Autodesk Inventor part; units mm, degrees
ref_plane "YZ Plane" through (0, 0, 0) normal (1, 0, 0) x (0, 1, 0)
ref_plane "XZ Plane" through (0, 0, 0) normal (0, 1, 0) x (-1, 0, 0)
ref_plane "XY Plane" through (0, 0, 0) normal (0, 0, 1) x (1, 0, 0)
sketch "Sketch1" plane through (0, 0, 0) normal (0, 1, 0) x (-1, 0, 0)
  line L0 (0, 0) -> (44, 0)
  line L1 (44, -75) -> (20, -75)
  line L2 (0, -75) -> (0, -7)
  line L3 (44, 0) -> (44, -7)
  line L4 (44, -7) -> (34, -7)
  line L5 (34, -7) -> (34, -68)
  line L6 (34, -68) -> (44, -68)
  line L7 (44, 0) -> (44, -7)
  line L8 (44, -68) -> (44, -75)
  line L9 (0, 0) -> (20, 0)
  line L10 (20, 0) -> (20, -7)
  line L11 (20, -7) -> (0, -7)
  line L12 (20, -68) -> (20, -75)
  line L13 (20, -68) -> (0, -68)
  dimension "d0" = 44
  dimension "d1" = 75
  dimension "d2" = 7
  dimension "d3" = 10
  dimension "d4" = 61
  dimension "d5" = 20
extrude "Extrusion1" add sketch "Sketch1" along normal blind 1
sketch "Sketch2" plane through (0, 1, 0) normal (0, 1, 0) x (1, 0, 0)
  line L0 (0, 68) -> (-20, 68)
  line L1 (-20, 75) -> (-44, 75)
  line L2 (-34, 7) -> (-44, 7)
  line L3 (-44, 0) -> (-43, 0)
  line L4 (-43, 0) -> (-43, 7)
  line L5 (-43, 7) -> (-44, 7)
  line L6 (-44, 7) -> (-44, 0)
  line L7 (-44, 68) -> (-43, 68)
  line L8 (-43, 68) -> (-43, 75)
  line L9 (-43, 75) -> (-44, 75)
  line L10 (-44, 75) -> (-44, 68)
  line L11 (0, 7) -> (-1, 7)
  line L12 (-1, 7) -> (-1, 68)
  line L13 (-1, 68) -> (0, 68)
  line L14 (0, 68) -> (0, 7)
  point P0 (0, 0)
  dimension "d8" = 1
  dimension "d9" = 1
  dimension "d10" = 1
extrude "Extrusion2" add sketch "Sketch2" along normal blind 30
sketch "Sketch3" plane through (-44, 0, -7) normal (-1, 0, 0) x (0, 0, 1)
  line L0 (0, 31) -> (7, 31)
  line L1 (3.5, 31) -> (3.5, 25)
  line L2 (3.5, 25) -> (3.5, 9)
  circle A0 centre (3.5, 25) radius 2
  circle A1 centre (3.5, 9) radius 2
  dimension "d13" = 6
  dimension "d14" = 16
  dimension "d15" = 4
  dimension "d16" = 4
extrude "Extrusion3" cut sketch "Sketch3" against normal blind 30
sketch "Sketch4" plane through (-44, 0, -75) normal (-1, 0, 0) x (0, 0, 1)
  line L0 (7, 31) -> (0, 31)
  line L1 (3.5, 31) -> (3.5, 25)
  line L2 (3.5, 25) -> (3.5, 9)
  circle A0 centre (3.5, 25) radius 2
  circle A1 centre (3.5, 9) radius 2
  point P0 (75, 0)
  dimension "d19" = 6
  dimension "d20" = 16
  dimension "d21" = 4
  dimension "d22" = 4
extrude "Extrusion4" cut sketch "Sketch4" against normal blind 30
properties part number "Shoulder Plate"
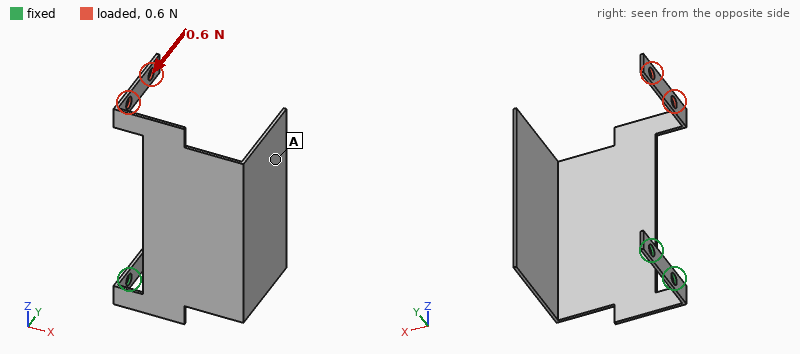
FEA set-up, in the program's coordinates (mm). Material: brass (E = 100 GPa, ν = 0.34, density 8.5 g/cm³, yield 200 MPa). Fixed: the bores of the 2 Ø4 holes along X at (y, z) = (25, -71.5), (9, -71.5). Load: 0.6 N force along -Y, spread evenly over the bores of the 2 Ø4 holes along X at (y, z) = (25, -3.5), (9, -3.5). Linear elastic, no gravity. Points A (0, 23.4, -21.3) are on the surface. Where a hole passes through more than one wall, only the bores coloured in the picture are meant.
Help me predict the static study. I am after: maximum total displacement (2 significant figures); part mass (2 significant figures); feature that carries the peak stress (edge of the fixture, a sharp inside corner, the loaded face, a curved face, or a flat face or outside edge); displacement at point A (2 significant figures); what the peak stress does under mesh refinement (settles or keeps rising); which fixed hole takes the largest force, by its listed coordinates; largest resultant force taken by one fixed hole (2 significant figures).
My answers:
0.85 mm
39 g
a sharp inside corner
0.49 mm
keeps rising
(9, -71.5)
0.65 N
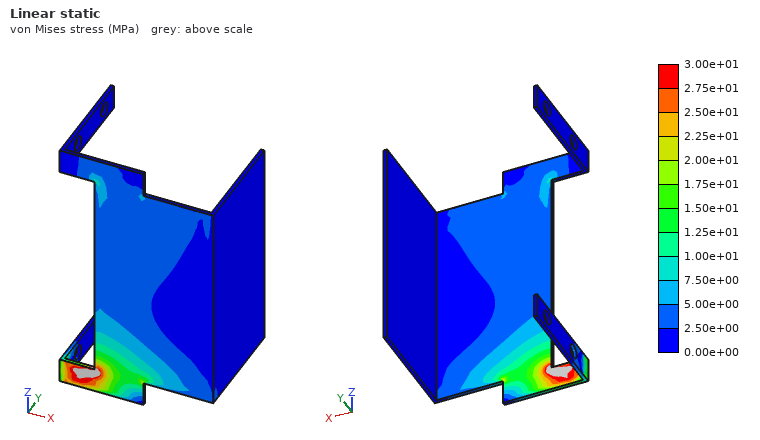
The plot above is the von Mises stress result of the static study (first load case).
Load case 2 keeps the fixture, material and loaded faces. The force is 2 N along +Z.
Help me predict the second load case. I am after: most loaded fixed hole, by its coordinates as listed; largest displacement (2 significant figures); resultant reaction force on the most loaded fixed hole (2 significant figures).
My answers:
(9, -71.5)
0.89 mm
1.9 N
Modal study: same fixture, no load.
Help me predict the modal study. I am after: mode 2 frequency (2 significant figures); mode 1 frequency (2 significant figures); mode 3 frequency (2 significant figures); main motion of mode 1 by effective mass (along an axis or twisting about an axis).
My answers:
54 Hz
32 Hz
80 Hz
along Y
